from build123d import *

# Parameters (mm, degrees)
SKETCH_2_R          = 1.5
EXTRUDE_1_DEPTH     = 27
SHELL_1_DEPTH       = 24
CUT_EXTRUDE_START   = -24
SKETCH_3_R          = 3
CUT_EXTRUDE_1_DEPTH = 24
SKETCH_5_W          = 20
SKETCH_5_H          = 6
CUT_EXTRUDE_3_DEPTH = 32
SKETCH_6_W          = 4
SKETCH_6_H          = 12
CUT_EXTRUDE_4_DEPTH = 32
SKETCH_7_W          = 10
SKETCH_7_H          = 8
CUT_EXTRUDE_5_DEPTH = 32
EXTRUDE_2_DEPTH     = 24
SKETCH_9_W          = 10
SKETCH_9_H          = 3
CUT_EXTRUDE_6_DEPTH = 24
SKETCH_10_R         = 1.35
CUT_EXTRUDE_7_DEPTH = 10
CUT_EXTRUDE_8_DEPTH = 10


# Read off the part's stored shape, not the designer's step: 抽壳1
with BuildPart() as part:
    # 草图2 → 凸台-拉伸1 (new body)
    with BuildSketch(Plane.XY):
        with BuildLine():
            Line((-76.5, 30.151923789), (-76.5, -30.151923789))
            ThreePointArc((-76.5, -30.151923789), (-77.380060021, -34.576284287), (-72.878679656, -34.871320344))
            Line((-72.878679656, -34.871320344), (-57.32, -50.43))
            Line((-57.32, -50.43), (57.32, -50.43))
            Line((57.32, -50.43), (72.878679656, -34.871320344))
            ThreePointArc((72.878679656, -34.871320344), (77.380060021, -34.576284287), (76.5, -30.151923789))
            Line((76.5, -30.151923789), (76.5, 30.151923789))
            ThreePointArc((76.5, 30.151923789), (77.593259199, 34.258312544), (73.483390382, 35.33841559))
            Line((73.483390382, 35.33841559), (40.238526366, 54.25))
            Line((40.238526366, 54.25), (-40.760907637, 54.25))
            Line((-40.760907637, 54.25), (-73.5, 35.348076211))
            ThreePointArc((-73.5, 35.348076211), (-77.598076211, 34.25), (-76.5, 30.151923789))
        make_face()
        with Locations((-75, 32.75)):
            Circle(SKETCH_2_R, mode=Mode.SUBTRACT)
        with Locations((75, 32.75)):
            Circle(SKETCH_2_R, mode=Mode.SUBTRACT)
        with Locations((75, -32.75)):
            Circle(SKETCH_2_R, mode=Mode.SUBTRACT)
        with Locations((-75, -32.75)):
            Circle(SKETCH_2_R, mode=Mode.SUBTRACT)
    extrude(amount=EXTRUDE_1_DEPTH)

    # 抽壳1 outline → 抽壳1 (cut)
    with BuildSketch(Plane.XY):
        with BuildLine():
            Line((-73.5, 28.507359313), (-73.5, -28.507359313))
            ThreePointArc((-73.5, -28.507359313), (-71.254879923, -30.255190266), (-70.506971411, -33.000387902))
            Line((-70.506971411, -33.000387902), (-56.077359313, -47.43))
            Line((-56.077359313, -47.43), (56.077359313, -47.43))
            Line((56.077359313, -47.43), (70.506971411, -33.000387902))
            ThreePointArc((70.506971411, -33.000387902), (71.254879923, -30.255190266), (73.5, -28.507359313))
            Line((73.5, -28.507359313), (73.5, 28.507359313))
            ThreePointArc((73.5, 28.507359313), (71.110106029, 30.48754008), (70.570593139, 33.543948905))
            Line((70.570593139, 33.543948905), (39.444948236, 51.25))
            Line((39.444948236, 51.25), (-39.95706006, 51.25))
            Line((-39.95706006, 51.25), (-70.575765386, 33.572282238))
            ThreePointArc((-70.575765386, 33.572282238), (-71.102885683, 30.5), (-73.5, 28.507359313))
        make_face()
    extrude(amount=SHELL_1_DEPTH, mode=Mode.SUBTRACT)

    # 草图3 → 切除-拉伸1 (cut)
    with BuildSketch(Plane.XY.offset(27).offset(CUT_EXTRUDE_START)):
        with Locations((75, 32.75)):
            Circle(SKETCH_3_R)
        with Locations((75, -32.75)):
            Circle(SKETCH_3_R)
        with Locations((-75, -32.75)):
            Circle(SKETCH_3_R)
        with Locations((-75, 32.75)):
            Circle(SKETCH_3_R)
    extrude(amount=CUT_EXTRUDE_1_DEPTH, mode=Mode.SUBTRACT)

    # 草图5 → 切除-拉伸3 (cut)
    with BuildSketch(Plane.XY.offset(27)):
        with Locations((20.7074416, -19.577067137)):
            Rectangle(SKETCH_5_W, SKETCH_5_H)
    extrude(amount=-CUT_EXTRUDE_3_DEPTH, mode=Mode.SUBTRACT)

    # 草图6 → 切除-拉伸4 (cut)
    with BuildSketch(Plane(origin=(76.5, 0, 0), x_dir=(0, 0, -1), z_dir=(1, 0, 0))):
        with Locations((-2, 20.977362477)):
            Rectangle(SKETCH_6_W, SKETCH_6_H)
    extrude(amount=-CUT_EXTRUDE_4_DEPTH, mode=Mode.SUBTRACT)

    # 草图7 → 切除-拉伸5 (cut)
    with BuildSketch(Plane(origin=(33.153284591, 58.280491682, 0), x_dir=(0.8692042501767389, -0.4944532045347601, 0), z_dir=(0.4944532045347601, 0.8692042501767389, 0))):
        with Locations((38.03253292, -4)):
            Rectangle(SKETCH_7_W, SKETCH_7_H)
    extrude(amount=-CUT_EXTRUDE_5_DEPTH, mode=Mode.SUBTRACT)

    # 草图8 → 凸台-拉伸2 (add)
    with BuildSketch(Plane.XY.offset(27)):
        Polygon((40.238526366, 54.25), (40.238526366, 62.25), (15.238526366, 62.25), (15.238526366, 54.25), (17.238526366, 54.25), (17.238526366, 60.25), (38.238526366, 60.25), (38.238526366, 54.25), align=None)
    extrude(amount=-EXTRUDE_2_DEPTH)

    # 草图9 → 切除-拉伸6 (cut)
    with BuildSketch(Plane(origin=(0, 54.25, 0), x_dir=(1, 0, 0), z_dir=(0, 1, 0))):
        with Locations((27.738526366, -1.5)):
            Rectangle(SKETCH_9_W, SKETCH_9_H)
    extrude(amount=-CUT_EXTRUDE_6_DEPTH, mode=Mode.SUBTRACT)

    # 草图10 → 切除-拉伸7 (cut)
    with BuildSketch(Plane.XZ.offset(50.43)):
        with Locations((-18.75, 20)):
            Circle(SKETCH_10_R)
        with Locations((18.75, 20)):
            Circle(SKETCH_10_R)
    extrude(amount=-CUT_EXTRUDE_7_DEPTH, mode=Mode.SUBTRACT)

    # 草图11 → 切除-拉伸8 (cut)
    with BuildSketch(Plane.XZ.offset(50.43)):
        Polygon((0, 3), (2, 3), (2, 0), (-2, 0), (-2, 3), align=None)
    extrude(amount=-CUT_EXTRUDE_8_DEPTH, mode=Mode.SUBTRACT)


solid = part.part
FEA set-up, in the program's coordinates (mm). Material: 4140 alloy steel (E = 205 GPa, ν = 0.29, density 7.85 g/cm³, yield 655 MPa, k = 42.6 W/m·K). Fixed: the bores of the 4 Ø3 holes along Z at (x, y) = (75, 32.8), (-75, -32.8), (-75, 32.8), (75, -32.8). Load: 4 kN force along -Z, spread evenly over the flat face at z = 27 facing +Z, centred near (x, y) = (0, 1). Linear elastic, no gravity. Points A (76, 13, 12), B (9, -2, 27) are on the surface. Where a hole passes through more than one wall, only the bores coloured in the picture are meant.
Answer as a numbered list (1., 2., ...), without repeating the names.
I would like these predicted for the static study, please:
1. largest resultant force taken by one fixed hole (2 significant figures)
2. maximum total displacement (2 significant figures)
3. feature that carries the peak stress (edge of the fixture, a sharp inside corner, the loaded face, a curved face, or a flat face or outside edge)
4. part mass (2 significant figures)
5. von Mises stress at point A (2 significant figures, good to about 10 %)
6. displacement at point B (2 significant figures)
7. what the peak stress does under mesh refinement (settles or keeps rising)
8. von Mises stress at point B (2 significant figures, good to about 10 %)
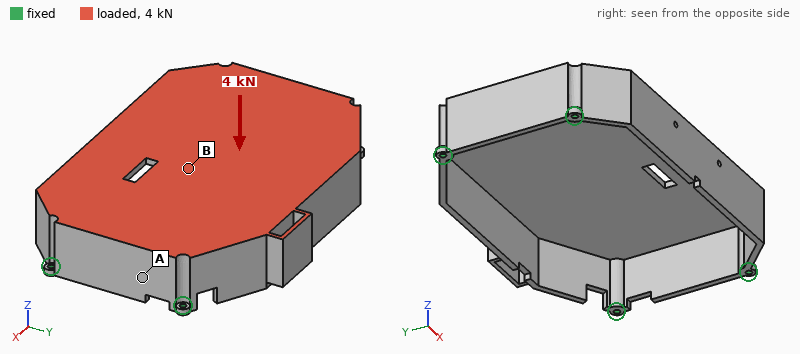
1. 1.2 kN
2. 0.23 mm
3. edge of the fixture
4. 610 g
5. 24 MPa
6. 0.23 mm
7. keeps rising
8. 75 MPa
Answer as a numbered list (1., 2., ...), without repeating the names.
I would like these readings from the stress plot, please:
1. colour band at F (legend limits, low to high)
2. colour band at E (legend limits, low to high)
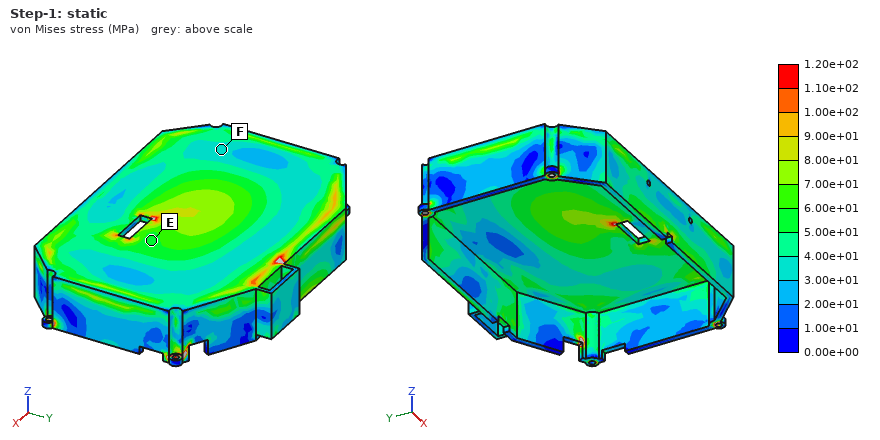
1. 3.00e+01 to 4.00e+01 MPa
2. 5.00e+01 to 6.00e+01 MPa
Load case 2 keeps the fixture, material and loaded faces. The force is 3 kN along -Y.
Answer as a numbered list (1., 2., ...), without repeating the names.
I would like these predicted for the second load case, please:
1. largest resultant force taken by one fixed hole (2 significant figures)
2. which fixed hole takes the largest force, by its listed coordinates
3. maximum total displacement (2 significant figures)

1. 1.1 kN
2. (75, -32.8)
3. 14 µm
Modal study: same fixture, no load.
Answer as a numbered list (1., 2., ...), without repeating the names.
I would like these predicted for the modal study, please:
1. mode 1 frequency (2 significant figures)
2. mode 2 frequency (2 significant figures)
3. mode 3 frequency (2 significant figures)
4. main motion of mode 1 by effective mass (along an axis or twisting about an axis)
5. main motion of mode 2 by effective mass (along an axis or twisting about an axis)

1. 1400 Hz
2. 1700 Hz
3. 2400 Hz
4. along Z
5. along X
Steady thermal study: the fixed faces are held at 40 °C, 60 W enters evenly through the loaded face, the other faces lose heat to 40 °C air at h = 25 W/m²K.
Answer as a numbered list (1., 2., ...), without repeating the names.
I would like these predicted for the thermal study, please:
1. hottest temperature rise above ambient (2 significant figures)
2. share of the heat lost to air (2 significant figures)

1. 67 K
2. 72 %
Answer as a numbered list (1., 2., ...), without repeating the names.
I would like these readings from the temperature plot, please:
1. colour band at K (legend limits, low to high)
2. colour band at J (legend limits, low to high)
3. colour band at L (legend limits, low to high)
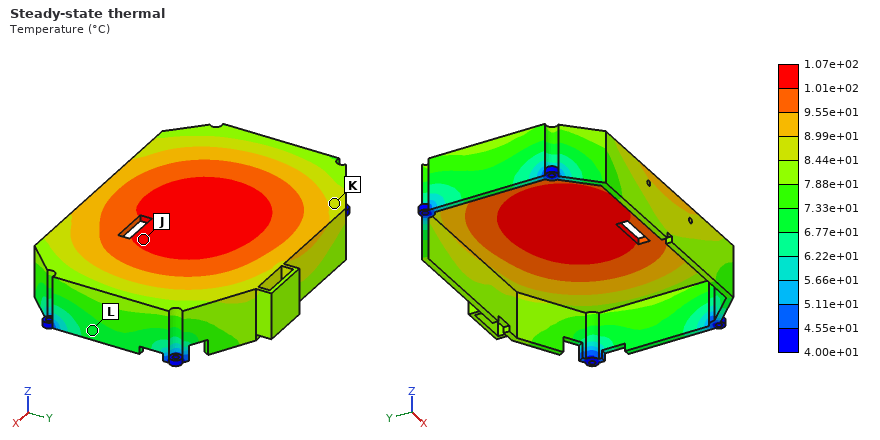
1. 8.44e+01 to 8.99e+01 °C
2. 1.01e+02 to 1.07e+02 °C
3. 6.77e+01 to 7.33e+01 °C
